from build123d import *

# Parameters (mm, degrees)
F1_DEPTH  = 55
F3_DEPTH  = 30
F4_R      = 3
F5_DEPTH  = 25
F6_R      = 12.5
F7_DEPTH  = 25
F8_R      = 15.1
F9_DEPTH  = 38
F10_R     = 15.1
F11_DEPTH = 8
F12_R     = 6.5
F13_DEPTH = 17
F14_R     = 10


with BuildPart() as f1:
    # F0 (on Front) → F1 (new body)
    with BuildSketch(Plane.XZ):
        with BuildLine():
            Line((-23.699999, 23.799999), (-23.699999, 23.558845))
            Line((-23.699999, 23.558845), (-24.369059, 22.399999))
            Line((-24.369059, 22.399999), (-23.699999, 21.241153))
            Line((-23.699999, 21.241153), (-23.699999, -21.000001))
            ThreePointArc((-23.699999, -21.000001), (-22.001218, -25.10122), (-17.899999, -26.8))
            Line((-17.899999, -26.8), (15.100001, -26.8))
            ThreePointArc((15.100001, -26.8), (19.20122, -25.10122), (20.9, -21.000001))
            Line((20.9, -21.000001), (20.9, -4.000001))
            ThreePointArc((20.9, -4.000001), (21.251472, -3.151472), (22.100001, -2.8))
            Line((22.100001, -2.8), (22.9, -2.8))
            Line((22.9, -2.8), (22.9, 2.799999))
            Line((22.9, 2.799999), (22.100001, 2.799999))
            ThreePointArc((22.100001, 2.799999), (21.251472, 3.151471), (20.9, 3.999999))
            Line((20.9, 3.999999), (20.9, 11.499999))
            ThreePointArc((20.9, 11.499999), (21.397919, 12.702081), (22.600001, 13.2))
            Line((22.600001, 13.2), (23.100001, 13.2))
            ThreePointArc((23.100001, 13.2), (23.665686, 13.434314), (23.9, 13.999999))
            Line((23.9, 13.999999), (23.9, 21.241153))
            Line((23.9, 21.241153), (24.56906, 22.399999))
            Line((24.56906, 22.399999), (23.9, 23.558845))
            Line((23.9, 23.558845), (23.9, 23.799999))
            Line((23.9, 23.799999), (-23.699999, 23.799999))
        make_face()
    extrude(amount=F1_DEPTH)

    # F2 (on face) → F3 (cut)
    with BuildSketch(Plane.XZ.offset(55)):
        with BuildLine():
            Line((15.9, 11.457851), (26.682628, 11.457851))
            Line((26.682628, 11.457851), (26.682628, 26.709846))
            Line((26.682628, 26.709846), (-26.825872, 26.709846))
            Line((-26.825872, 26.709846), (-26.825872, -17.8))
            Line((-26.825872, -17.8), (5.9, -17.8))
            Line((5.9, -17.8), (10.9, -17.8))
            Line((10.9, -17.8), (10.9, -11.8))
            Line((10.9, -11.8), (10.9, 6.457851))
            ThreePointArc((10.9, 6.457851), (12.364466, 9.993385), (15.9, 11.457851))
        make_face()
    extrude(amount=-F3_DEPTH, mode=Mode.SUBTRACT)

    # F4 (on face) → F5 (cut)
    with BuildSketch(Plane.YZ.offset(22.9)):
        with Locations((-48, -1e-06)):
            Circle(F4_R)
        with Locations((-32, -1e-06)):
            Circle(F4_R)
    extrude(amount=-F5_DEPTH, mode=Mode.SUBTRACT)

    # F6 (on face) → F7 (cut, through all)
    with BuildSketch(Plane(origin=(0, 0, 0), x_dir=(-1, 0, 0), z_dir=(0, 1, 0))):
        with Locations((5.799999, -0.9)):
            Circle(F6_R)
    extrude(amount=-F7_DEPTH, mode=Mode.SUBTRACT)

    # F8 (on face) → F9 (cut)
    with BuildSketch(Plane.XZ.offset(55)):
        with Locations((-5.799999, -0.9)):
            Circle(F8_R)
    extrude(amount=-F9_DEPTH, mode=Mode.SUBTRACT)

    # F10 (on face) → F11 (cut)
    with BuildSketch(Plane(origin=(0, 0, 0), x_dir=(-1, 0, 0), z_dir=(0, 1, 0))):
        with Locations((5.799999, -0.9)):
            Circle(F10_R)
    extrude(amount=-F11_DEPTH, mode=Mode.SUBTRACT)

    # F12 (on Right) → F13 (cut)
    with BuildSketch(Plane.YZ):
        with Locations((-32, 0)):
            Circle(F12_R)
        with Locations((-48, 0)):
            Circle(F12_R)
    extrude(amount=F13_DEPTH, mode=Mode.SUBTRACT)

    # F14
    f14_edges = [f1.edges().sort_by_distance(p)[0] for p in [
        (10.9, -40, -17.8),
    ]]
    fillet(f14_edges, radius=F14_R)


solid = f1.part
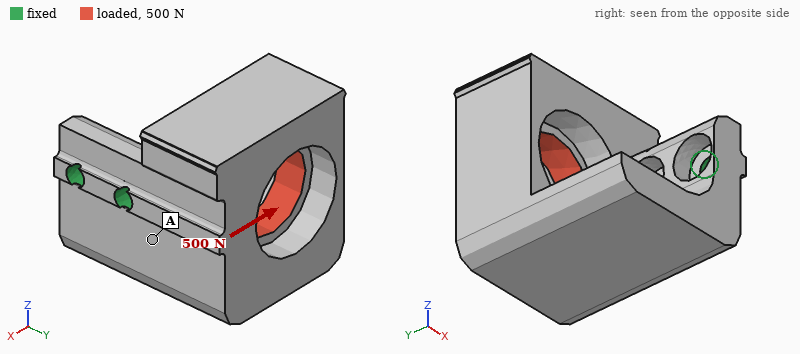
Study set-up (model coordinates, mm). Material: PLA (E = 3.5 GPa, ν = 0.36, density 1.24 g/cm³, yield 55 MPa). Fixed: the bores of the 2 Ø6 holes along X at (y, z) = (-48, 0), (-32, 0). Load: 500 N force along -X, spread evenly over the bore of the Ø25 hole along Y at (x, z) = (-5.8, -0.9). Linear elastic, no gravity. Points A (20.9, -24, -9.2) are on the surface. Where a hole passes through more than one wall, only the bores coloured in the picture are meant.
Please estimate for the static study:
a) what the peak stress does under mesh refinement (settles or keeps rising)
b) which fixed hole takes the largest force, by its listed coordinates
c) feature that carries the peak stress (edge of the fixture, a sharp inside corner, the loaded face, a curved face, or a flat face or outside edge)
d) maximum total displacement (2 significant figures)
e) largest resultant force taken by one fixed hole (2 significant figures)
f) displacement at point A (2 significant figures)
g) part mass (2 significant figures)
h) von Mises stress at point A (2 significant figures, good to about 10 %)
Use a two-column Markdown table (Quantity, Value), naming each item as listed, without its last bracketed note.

| Quantity | Value |
|---|---|
| what the peak stress does under mesh refinement | keeps rising |
| which fixed hole takes the largest force, by its listed coordinates | (-32, 0) |
| feature that carries the peak stress | edge of the fixture |
| maximum total displacement | 0.57 mm |
| largest resultant force taken by one fixed hole | 860 N |
| displacement at point A | 0.12 mm |
| part mass | 75 g |
| von Mises stress at point A | 3.4 MPa |
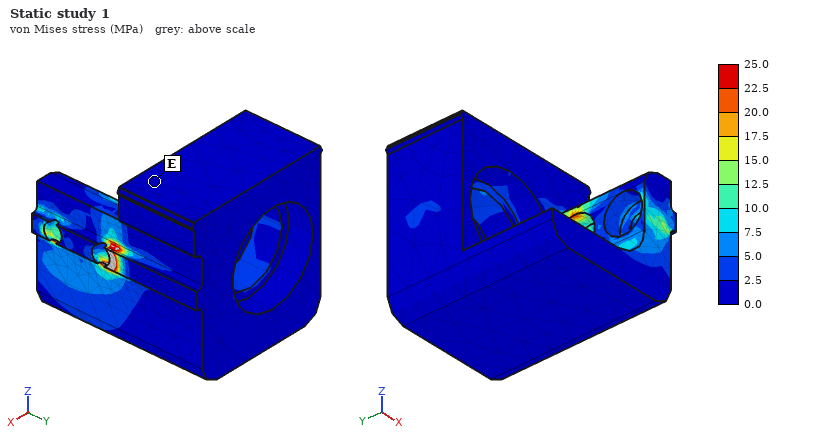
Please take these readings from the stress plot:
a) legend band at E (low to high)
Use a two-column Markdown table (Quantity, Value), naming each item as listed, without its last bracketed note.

| Quantity | Value |
|---|---|
| legend band at E | 0.0 to 2.5 MPa |
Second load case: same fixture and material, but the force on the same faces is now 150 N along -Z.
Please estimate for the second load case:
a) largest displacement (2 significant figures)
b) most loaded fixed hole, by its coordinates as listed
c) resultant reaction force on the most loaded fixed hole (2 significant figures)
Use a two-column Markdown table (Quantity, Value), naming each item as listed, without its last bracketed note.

| Quantity | Value |
|---|---|
| largest displacement | 0.48 mm |
| most loaded fixed hole, by its coordinates as listed | (-32, 0) |
| resultant reaction force on the most loaded fixed hole | 260 N |
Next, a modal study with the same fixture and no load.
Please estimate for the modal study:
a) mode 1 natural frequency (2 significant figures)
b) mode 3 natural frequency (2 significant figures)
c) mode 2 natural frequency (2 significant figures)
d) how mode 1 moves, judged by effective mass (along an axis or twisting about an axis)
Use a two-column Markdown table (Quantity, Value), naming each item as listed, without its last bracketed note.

| Quantity | Value |
|---|---|
| mode 1 natural frequency | 430 Hz |
| mode 3 natural frequency | 1300 Hz |
| mode 2 natural frequency | 670 Hz |
| how mode 1 moves, judged by effective mass | along Z |
